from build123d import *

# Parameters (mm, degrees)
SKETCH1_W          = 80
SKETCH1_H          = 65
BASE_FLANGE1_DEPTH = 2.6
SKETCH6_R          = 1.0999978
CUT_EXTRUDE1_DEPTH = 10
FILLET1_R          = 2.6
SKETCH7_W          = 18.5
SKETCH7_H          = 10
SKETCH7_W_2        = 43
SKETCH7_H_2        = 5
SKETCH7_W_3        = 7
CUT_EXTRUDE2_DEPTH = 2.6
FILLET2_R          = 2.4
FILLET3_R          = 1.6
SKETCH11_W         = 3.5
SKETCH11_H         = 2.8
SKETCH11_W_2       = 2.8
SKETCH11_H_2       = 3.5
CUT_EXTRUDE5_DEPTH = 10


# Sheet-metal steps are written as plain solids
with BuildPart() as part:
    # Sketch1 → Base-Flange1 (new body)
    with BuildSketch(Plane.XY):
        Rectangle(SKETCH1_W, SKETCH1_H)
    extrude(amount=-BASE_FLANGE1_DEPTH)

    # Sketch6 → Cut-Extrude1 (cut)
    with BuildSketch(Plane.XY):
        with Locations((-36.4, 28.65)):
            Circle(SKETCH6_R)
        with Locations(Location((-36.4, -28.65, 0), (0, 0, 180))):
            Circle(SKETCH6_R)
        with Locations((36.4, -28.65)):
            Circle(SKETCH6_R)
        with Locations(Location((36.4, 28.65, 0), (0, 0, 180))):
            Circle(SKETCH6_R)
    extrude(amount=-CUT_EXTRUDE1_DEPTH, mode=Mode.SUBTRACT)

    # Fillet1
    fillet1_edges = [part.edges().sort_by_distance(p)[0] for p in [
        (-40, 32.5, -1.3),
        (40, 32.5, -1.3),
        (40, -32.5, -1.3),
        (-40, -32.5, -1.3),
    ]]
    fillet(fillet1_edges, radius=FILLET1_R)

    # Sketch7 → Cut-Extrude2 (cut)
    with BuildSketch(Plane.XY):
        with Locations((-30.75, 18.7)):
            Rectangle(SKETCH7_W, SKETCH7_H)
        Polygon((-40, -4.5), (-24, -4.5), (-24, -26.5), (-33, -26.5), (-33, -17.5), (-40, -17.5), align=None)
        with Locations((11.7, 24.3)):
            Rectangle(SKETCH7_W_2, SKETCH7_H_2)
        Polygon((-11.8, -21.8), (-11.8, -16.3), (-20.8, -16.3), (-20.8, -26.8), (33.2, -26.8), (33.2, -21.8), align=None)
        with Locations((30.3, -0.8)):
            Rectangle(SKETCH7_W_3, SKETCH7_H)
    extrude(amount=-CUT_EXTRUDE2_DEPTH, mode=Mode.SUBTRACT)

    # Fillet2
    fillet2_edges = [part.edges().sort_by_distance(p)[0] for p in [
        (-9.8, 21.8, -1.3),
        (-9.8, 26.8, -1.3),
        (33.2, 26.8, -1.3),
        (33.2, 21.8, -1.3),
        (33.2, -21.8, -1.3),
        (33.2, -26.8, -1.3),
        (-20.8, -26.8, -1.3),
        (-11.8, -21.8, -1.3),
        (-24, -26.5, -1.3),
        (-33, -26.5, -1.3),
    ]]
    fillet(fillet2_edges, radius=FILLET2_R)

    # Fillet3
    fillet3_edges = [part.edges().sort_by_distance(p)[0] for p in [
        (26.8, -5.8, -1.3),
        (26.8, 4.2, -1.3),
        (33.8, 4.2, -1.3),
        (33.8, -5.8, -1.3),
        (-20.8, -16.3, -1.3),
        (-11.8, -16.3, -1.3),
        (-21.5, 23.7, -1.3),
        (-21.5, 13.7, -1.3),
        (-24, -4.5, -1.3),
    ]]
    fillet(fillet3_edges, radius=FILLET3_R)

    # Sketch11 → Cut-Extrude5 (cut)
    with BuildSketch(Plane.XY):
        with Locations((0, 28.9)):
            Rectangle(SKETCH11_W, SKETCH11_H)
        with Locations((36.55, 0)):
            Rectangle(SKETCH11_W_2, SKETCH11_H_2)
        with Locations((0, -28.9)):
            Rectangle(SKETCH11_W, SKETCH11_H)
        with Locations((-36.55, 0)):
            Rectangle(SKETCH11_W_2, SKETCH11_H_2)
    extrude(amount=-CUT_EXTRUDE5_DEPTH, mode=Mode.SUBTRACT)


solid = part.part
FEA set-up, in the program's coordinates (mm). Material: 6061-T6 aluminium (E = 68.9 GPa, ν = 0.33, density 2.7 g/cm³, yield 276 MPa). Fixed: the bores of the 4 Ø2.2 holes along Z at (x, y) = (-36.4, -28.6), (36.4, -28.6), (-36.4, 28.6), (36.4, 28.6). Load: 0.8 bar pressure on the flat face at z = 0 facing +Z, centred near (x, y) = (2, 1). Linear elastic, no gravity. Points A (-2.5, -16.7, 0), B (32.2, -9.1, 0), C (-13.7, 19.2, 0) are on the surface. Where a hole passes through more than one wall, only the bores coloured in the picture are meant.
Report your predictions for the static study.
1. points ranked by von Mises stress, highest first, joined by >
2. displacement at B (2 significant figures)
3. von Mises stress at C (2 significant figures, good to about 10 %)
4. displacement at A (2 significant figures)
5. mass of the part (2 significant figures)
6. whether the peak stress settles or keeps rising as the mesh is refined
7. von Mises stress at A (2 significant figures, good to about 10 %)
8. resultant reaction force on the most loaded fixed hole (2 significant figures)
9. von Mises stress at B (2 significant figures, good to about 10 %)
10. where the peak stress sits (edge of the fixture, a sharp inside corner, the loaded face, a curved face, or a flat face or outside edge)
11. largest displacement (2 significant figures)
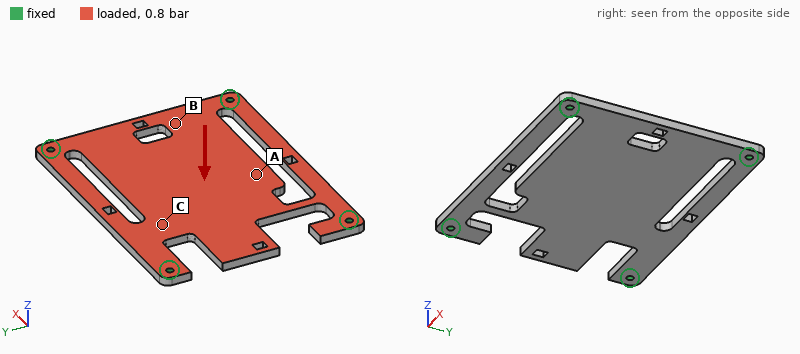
C > A > B
0.062 mm
28 MPa
0.18 mm
29 g
keeps rising
19 MPa
88 N
8.2 MPa
edge of the fixture
0.21 mm
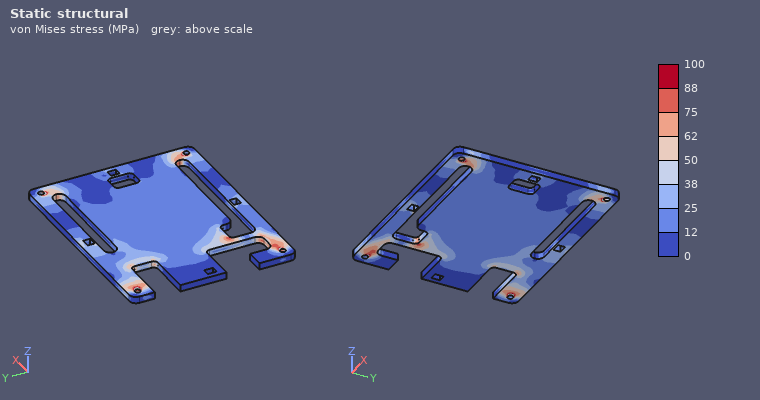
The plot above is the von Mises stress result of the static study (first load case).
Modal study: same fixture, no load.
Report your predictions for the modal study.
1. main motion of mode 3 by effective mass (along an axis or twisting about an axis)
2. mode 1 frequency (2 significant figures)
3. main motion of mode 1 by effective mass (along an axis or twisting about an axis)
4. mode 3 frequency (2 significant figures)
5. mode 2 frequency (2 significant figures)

twisting about X
1400 Hz
along Z
2700 Hz
2200 Hz
